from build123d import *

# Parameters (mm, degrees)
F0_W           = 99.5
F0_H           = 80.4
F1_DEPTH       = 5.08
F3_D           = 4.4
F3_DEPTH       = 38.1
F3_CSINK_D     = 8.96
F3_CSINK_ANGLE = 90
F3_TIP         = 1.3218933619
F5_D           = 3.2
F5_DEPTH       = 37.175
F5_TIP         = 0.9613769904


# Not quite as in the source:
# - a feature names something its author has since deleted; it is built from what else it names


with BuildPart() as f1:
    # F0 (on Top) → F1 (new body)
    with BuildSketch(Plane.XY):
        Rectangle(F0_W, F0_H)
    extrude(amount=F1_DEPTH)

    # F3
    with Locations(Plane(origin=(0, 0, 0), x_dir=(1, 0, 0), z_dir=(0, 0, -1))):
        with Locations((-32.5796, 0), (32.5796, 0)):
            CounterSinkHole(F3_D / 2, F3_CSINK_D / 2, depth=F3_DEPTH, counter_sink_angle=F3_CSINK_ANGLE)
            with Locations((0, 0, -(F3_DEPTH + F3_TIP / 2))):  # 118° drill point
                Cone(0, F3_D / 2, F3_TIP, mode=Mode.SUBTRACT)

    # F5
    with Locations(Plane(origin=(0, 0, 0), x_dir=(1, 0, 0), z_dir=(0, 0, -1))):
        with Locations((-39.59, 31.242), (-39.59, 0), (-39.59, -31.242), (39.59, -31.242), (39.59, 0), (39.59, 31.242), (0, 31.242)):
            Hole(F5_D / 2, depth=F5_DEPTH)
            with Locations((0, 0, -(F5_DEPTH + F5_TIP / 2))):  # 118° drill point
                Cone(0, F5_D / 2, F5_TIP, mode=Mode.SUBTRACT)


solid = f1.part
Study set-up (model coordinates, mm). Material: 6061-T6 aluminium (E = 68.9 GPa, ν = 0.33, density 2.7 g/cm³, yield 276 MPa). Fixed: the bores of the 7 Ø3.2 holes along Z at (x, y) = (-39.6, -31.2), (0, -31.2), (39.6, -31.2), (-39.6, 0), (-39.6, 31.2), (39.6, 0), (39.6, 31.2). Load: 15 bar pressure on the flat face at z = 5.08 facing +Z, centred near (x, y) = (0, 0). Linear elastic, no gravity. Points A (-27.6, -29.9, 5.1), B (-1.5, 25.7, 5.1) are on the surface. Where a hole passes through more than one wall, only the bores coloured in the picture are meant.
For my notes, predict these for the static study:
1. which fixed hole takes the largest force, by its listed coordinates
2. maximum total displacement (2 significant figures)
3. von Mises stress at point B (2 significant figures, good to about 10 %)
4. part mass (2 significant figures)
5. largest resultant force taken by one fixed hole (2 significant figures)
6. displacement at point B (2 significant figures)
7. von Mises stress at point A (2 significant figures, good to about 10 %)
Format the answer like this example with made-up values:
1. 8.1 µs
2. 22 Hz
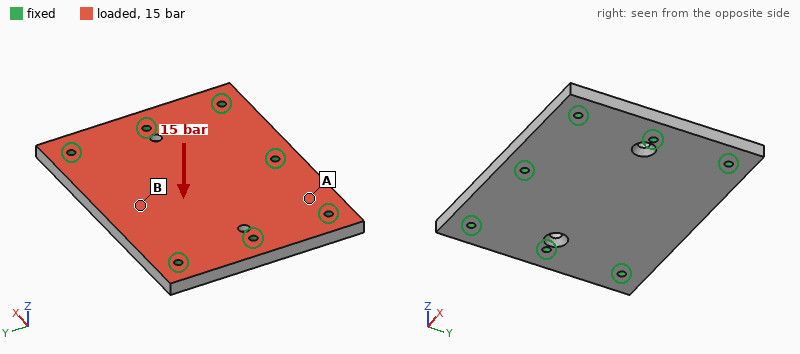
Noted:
1. (0, -31.2)
2. 0.27 mm
3. 84 MPa
4. 110 g
5. 2.4 kN
6. 0.23 mm
7. 26 MPa
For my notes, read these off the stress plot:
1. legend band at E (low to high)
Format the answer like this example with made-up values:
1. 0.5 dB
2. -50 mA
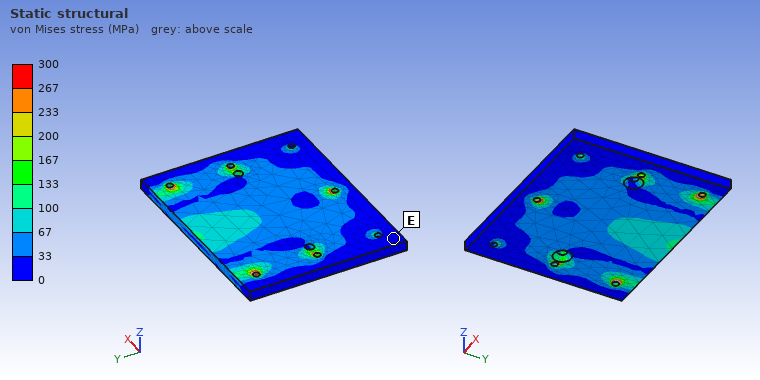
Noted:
1. 0 to 33 MPa
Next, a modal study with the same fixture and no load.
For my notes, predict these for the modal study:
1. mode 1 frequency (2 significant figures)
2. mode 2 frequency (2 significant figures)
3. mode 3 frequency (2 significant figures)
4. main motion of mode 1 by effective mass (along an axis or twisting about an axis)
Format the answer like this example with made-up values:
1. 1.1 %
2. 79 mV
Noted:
1. 4100 Hz
2. 7400 Hz
3. 10 kHz
4. along Z
